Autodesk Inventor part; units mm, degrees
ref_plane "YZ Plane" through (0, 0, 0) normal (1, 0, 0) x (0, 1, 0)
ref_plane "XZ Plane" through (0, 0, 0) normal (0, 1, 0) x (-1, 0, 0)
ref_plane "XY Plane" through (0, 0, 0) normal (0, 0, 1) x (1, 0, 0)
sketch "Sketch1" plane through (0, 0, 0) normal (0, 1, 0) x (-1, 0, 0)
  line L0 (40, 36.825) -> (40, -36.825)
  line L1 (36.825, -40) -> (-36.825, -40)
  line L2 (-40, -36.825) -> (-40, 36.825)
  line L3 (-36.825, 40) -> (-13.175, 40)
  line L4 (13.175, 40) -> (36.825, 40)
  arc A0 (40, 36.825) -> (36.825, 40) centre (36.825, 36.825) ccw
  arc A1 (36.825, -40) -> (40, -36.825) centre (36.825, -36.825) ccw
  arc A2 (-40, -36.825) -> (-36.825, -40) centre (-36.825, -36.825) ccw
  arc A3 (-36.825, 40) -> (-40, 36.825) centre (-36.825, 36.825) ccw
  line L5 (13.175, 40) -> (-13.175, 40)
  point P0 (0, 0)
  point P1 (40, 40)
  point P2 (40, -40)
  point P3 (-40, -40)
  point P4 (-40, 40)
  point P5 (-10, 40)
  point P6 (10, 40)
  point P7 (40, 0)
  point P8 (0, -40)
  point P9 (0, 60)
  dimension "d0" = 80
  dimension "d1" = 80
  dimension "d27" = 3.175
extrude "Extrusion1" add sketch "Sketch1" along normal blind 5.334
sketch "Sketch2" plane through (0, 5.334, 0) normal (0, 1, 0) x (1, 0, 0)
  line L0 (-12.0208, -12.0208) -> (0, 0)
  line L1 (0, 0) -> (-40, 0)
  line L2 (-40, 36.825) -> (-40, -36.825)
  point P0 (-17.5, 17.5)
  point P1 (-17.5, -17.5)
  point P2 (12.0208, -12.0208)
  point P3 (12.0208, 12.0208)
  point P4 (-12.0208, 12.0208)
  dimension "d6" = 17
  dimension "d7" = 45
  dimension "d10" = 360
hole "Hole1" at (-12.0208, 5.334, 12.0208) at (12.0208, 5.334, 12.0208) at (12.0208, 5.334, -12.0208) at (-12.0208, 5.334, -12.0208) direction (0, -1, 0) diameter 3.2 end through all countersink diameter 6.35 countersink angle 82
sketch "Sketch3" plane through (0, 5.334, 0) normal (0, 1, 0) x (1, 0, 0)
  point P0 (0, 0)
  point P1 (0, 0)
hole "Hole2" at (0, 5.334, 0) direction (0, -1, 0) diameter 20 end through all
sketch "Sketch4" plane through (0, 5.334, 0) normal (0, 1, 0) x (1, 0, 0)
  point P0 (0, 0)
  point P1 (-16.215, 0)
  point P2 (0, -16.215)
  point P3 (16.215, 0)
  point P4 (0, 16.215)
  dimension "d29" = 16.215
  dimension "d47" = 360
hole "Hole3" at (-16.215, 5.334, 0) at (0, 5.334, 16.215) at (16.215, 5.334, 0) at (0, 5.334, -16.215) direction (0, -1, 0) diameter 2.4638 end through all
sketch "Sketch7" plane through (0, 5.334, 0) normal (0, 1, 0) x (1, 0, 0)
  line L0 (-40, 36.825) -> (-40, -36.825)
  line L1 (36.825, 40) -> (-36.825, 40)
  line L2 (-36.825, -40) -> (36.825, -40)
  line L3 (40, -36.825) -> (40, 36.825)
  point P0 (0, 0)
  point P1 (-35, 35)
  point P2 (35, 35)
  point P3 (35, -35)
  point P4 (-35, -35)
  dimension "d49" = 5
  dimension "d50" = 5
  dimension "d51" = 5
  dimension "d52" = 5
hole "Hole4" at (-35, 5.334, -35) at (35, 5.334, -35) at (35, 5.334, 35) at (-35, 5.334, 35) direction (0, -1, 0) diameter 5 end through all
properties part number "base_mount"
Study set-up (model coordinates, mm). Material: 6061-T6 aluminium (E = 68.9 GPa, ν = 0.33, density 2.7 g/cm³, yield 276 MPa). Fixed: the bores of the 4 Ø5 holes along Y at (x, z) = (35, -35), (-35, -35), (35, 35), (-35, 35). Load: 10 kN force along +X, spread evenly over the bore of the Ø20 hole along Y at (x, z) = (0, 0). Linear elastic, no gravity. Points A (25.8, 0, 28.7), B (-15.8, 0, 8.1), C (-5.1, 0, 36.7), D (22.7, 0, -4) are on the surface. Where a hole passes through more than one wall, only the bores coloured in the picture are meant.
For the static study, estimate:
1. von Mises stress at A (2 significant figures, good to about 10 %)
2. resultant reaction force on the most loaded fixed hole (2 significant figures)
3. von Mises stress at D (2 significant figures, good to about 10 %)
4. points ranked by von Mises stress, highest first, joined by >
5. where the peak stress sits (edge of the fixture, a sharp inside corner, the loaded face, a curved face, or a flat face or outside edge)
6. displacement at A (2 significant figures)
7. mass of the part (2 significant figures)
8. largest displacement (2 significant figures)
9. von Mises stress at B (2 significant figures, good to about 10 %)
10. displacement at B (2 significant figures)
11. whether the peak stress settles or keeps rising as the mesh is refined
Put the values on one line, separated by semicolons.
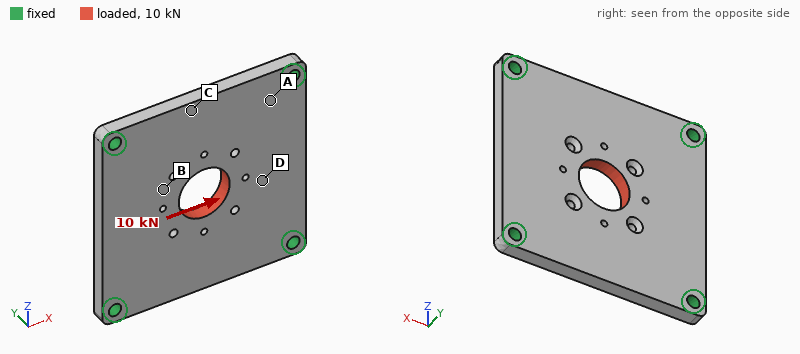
32 MPa; 2.8 kN; 14 MPa; A > B > D > C; edge of the fixture; 6.3 µm; 85 g; 24 µm; 22 MPa; 19 µm; keeps rising
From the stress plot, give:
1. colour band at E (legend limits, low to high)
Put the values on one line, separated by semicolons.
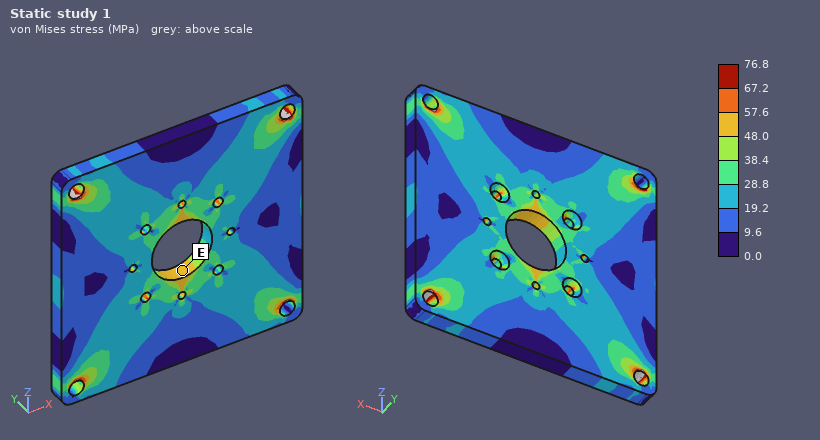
48.0 to 57.6 MPa
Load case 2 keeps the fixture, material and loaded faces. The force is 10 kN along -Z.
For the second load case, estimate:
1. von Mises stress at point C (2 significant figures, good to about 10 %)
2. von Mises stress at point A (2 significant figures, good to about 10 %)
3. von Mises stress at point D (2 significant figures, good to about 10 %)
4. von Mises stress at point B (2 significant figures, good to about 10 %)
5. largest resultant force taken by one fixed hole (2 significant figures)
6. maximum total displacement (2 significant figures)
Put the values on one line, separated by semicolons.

13 MPa; 30 MPa; 18 MPa; 24 MPa; 2.8 kN; 24 µm
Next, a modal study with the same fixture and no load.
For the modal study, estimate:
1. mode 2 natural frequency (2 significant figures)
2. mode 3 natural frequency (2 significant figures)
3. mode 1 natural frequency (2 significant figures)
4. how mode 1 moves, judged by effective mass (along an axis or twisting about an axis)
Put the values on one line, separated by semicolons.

6100 Hz; 6100 Hz; 3600 Hz; along Y
